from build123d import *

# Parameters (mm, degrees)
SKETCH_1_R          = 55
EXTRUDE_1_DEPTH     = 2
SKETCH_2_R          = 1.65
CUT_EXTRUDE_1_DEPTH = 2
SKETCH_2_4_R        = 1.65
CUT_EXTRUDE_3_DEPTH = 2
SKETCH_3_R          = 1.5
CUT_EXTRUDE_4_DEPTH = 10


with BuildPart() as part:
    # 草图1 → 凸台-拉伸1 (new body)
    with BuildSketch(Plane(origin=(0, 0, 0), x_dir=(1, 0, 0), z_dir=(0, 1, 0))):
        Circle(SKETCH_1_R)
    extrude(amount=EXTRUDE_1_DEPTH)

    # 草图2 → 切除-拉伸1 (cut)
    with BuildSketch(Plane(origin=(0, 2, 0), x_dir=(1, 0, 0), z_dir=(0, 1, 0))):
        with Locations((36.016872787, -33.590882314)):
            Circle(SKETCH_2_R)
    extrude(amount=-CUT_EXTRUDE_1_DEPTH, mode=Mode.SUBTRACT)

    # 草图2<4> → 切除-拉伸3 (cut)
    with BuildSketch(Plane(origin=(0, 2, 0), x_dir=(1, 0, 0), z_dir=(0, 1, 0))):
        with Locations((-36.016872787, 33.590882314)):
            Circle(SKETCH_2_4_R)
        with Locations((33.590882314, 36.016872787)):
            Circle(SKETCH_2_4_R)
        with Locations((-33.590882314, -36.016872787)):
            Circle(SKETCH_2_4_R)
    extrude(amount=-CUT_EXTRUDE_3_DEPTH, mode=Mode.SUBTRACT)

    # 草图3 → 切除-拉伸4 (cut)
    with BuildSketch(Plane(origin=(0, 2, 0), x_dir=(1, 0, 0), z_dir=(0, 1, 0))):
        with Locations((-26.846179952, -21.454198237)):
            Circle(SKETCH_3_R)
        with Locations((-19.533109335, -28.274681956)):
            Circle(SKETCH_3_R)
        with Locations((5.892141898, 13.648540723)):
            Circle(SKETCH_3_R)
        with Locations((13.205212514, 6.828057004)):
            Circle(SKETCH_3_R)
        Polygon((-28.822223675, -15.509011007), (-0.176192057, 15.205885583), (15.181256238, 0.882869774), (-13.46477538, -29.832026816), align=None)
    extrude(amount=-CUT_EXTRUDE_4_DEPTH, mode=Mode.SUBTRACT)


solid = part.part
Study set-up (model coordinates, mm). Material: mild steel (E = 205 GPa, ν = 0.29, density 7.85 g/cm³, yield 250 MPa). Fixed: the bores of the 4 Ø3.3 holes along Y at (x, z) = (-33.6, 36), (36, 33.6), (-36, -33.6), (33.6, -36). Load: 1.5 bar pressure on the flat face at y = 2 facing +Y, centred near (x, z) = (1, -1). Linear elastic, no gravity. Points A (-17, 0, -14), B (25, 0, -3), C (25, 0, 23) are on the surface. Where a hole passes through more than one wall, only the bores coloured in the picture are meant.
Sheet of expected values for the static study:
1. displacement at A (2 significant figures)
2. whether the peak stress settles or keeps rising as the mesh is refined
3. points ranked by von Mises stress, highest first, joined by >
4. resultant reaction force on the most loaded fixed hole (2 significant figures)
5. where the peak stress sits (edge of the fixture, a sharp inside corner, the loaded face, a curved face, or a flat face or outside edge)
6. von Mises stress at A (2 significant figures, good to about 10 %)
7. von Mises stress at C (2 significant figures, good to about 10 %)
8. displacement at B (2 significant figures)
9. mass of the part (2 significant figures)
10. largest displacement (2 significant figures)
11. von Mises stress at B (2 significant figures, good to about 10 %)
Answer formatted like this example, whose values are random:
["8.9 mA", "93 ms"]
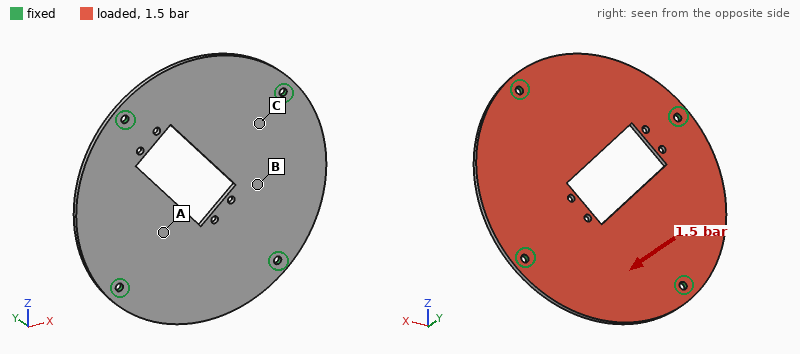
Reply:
["0.11 mm", "keeps rising", "B > C > A", "330 N", "edge of the fixture", "18 MPa", "35 MPa", "0.12 mm", "130 g", "0.16 mm", "56 MPa"]
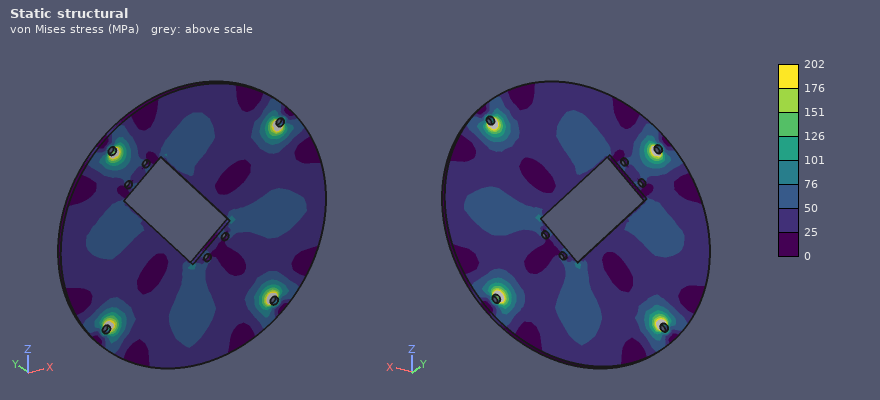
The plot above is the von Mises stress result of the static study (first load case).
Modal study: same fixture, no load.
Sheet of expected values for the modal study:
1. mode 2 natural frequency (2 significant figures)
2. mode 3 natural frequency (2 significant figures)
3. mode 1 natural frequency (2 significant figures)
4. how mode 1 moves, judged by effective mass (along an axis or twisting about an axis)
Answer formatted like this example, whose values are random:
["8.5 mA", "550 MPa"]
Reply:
["1700 Hz", "1800 Hz", "1600 Hz", "along Y"]
